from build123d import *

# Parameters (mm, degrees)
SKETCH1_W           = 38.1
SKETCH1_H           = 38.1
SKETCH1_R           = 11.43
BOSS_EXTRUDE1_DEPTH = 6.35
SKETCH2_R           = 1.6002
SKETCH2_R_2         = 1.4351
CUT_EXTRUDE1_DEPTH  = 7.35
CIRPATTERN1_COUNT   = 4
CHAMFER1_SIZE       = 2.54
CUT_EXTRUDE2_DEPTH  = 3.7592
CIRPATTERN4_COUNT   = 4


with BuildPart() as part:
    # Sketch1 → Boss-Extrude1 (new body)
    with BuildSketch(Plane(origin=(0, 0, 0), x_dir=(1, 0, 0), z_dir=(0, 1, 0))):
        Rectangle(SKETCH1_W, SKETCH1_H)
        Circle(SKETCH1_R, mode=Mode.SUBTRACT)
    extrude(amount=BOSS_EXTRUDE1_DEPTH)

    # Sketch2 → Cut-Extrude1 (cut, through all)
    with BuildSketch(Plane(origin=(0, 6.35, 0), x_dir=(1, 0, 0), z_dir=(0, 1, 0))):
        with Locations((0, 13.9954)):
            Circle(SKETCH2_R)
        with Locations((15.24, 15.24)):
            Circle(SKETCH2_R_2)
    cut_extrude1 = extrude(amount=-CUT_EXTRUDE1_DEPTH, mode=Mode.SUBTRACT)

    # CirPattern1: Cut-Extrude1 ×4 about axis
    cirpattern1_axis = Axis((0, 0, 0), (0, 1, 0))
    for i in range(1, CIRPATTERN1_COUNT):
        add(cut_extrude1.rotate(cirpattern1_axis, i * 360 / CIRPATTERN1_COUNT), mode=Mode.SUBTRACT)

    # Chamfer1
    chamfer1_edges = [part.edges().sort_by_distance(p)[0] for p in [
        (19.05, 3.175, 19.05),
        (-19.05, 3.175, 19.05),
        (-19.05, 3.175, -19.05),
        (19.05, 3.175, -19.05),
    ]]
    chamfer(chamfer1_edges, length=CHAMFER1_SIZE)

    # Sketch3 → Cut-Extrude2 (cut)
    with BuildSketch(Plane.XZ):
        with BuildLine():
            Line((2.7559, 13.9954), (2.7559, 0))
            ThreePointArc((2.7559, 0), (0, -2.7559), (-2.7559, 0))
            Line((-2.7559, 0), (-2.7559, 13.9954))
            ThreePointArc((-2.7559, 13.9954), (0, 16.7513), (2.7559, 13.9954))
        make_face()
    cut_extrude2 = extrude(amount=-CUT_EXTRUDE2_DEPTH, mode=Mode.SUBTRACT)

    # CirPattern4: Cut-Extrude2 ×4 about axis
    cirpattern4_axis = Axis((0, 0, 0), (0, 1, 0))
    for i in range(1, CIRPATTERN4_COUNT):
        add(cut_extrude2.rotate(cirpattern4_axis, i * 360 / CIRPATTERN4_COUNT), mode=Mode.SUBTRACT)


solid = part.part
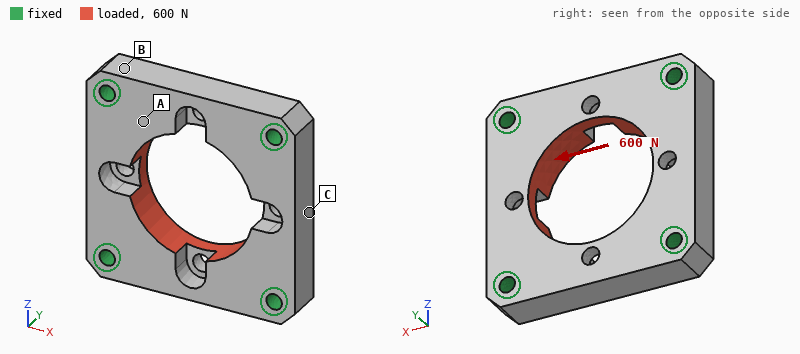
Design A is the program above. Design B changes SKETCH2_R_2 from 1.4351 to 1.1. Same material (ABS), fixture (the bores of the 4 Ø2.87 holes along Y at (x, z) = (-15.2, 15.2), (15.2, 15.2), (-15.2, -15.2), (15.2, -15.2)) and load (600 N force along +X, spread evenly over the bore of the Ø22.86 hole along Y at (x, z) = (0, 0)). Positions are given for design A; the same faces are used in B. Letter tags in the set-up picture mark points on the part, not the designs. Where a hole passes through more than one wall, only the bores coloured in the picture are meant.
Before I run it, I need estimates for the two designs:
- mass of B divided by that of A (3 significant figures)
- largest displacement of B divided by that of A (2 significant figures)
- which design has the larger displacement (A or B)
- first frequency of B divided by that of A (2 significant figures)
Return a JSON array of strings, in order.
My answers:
["1.01", "1.1", "B", "0.89"]
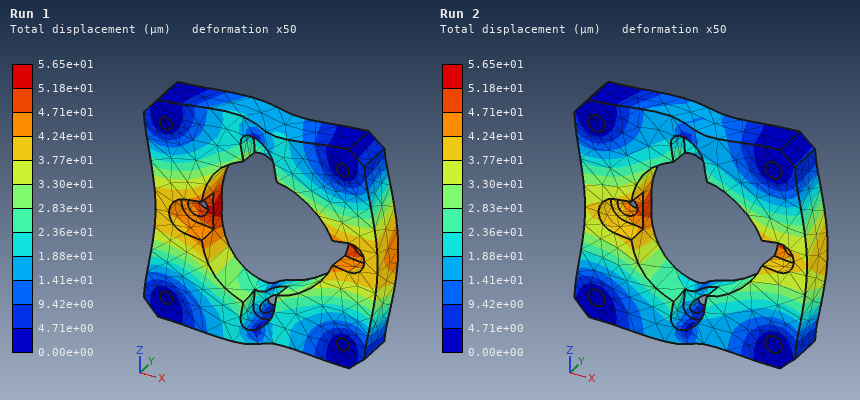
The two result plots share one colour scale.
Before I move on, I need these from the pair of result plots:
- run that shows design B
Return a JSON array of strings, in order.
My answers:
["Run 1"]
